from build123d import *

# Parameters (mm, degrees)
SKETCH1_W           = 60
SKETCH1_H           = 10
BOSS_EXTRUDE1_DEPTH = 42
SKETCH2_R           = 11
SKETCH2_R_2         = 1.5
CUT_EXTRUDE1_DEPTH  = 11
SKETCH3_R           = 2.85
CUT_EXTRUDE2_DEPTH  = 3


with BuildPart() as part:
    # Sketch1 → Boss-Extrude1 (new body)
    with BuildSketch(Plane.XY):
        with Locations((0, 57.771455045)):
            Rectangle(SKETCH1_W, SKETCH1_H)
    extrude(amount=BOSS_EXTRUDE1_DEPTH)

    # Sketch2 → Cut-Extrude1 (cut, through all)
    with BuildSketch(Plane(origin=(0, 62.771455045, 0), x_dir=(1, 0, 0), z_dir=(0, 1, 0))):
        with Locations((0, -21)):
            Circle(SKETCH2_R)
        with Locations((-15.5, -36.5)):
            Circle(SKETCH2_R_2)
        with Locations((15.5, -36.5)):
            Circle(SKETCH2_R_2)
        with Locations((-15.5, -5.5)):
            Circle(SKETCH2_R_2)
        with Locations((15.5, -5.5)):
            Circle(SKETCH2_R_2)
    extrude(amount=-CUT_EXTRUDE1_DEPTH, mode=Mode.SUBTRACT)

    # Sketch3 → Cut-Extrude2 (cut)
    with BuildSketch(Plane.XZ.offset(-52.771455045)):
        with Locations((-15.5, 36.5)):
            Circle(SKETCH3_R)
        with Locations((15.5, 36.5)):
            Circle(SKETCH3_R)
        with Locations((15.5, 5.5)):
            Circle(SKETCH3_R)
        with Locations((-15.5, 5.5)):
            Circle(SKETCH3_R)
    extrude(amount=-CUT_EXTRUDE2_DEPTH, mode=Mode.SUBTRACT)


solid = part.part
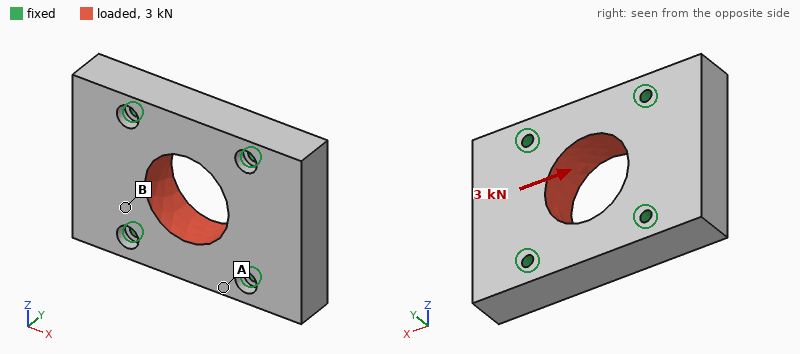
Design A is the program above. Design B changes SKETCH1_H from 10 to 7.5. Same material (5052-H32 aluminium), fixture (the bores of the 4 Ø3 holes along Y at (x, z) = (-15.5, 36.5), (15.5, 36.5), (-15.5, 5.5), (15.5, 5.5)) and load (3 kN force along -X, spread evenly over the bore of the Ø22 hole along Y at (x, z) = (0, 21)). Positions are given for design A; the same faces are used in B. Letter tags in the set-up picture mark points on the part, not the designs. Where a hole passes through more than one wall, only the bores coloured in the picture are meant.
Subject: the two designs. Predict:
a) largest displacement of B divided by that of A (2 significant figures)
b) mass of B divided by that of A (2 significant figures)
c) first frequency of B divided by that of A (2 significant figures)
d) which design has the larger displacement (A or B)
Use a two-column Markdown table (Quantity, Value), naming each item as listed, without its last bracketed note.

| Quantity | Value |
|---|---|
| largest displacement of B divided by that of A | 1.2 |
| mass of B divided by that of A | 0.75 |
| first frequency of B divided by that of A | 0.89 |
| which design has the larger displacement | B |
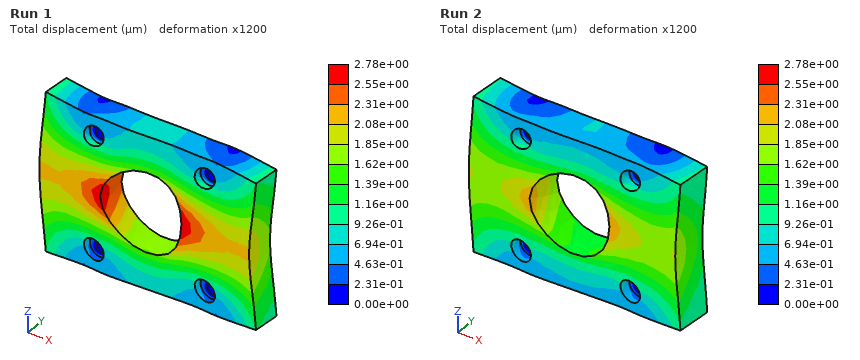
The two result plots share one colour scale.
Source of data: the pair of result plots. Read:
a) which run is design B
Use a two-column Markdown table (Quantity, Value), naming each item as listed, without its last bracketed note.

| Quantity | Value |
|---|---|
| which run is design B | Run 1 |
